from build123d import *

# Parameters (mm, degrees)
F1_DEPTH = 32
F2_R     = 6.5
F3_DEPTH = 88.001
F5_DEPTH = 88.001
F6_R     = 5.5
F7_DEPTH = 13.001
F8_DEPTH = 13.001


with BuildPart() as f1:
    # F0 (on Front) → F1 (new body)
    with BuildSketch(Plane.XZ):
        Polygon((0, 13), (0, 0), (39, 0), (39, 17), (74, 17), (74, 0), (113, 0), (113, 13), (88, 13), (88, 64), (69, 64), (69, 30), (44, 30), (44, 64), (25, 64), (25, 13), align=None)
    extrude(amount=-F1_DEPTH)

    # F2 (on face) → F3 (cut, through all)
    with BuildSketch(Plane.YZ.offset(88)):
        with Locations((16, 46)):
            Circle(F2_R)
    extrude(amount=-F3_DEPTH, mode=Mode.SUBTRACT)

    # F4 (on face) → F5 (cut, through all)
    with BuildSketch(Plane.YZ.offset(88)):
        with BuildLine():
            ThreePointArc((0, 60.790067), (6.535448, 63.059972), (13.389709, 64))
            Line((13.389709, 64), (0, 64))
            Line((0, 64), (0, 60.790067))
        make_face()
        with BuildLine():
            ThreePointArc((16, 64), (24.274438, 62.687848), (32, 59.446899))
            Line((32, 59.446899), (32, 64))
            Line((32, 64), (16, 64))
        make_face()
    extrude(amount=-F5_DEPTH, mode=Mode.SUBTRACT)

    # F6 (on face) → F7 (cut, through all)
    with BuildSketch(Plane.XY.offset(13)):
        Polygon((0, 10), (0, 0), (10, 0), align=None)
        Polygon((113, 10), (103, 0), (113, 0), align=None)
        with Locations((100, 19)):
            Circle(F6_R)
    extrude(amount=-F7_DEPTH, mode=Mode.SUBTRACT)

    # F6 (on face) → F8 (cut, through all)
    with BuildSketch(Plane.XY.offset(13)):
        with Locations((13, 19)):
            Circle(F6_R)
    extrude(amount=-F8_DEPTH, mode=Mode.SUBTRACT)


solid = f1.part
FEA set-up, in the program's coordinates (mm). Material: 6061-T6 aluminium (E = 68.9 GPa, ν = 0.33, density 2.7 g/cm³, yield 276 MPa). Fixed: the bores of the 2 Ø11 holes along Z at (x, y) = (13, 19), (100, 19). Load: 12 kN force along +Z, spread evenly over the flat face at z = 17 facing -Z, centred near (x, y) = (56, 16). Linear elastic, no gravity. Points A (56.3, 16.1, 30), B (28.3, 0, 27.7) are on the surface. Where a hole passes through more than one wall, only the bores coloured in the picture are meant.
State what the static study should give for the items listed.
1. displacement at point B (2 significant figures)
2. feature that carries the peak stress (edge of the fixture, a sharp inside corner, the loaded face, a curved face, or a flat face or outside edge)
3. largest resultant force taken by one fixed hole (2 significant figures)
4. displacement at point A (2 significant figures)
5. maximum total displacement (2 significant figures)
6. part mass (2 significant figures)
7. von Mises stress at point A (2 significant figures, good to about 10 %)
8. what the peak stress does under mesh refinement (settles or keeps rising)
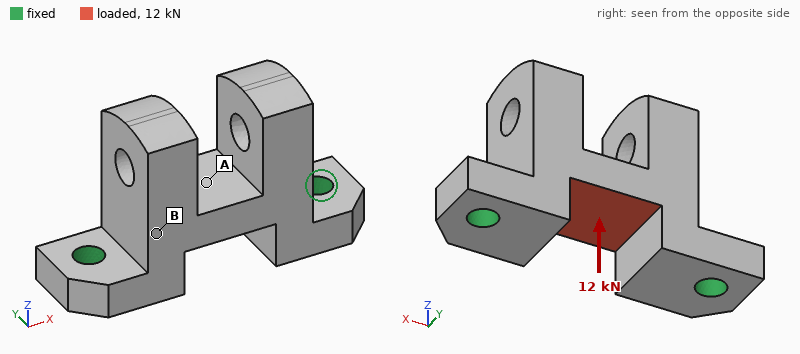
24 µm
edge of the fixture
8.6 kN
41 µm
58 µm
250 g
55 MPa
keeps rising
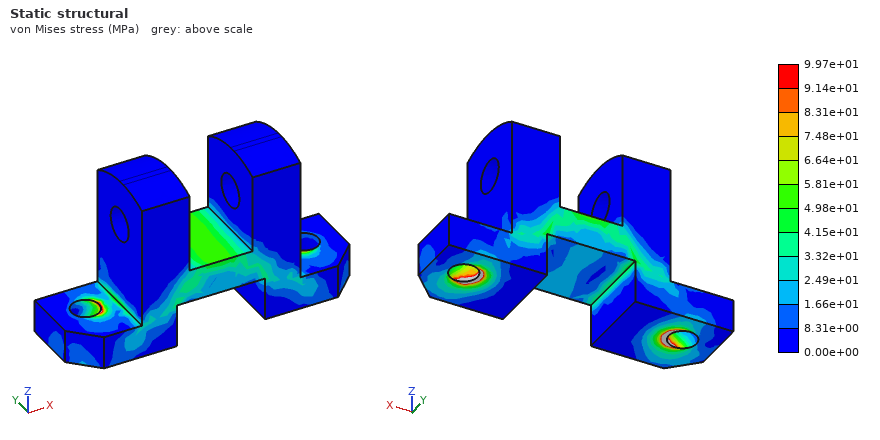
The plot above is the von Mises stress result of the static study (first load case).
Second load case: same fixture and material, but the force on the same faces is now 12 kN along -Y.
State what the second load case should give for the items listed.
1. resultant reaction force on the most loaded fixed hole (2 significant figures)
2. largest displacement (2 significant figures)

6.0 kN
0.13 mm
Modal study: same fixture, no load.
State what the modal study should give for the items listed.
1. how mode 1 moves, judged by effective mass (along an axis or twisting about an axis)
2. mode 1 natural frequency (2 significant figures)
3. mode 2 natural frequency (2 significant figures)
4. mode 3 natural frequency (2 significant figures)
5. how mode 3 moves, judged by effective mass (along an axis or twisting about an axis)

along Y
2800 Hz
4600 Hz
5700 Hz
along X
